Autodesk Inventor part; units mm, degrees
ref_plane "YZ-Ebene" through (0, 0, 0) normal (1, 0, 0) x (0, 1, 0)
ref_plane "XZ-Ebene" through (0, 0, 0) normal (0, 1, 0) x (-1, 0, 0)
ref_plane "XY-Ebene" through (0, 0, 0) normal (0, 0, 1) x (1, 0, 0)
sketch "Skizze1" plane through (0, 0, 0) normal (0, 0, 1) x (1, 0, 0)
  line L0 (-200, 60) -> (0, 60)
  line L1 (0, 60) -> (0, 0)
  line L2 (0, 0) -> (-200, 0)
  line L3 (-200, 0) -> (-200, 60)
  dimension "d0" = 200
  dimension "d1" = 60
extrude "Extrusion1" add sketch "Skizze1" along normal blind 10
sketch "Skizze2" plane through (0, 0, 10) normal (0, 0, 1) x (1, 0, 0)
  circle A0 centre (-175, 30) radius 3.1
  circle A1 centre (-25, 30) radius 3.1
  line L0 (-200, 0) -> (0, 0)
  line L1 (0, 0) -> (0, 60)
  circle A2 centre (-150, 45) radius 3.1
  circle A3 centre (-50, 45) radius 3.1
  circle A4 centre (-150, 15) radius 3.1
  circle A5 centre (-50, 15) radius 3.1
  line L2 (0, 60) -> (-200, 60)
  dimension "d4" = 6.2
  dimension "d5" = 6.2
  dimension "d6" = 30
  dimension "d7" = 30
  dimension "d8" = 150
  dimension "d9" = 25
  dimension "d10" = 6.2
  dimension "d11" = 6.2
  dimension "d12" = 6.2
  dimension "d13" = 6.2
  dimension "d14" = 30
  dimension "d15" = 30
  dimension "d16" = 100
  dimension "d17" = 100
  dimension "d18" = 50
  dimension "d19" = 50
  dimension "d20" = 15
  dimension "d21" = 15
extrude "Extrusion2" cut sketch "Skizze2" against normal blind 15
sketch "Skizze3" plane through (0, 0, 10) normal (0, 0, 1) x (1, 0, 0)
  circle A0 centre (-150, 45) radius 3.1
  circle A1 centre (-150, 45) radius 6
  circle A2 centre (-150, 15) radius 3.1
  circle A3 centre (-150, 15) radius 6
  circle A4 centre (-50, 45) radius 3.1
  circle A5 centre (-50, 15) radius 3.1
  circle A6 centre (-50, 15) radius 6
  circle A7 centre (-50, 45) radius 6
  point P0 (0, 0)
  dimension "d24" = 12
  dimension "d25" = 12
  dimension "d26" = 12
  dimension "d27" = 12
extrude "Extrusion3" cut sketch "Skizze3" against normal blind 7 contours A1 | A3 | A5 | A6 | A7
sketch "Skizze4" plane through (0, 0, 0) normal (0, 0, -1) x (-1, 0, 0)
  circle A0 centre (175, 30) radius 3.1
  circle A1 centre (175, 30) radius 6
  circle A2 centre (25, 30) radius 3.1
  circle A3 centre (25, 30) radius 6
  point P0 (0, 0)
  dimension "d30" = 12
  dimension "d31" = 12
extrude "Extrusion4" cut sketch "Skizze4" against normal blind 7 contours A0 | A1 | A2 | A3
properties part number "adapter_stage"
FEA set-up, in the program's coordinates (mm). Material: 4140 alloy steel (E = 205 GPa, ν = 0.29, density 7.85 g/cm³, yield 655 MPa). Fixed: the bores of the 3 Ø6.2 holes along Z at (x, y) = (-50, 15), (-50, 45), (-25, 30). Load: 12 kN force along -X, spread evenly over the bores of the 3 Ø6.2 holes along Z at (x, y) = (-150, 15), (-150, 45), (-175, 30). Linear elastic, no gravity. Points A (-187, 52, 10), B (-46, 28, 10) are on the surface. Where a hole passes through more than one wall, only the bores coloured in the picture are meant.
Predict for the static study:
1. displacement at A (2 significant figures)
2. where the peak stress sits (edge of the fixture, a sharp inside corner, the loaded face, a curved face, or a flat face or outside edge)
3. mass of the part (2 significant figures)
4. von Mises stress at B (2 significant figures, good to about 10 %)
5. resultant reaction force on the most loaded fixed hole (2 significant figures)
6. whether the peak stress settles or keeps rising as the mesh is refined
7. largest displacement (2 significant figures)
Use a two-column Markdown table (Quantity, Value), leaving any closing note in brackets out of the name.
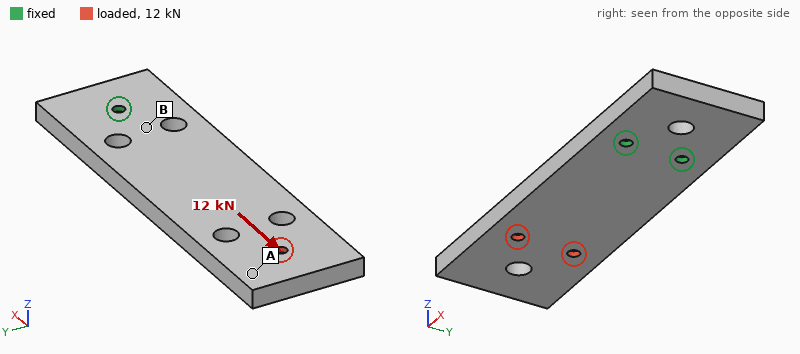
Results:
| Quantity | Value |
|---|---|
| displacement at A | 61 µm |
| where the peak stress sits | edge of the fixture |
| mass of the part | 900 g |
| von Mises stress at B | 23 MPa |
| resultant reaction force on the most loaded fixed hole | 4.6 kN |
| whether the peak stress settles or keeps rising as the mesh is refined | keeps rising |
| largest displacement | 70 µm |
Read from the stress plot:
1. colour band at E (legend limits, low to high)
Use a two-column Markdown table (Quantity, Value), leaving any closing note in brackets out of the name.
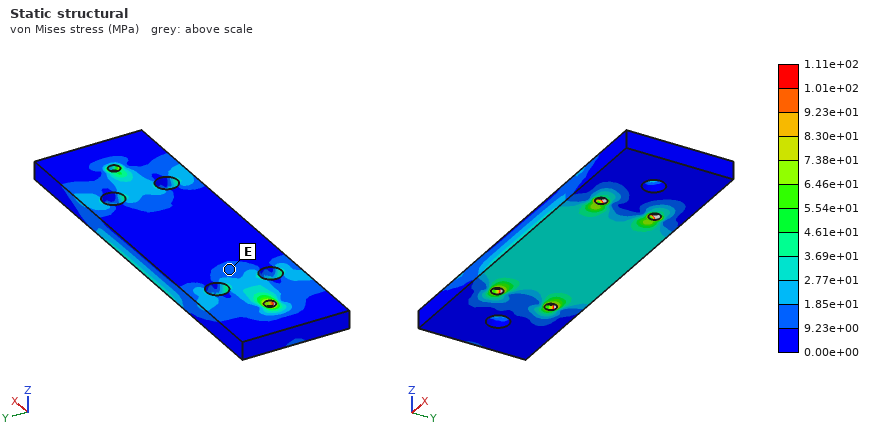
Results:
| Quantity | Value |
|---|---|
| colour band at E | 9.23e+00 to 1.85e+01 MPa |
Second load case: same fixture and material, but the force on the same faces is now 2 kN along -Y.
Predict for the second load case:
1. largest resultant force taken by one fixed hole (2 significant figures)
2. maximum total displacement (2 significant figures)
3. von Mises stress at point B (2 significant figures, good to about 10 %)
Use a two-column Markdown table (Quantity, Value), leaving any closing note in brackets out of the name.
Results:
| Quantity | Value |
|---|---|
| largest resultant force taken by one fixed hole | 5.3 kN |
| maximum total displacement | 74 µm |
| von Mises stress at point B | 18 MPa |
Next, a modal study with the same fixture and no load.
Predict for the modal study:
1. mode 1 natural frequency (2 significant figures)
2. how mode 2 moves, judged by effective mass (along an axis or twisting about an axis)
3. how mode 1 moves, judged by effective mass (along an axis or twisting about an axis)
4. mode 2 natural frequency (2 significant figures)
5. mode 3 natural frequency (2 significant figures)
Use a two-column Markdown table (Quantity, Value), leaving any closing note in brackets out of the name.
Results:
| Quantity | Value |
|---|---|
| mode 1 natural frequency | 330 Hz |
| how mode 2 moves, judged by effective mass | along Y |
| how mode 1 moves, judged by effective mass | along Z |
| mode 2 natural frequency | 1500 Hz |
| mode 3 natural frequency | 1700 Hz |
